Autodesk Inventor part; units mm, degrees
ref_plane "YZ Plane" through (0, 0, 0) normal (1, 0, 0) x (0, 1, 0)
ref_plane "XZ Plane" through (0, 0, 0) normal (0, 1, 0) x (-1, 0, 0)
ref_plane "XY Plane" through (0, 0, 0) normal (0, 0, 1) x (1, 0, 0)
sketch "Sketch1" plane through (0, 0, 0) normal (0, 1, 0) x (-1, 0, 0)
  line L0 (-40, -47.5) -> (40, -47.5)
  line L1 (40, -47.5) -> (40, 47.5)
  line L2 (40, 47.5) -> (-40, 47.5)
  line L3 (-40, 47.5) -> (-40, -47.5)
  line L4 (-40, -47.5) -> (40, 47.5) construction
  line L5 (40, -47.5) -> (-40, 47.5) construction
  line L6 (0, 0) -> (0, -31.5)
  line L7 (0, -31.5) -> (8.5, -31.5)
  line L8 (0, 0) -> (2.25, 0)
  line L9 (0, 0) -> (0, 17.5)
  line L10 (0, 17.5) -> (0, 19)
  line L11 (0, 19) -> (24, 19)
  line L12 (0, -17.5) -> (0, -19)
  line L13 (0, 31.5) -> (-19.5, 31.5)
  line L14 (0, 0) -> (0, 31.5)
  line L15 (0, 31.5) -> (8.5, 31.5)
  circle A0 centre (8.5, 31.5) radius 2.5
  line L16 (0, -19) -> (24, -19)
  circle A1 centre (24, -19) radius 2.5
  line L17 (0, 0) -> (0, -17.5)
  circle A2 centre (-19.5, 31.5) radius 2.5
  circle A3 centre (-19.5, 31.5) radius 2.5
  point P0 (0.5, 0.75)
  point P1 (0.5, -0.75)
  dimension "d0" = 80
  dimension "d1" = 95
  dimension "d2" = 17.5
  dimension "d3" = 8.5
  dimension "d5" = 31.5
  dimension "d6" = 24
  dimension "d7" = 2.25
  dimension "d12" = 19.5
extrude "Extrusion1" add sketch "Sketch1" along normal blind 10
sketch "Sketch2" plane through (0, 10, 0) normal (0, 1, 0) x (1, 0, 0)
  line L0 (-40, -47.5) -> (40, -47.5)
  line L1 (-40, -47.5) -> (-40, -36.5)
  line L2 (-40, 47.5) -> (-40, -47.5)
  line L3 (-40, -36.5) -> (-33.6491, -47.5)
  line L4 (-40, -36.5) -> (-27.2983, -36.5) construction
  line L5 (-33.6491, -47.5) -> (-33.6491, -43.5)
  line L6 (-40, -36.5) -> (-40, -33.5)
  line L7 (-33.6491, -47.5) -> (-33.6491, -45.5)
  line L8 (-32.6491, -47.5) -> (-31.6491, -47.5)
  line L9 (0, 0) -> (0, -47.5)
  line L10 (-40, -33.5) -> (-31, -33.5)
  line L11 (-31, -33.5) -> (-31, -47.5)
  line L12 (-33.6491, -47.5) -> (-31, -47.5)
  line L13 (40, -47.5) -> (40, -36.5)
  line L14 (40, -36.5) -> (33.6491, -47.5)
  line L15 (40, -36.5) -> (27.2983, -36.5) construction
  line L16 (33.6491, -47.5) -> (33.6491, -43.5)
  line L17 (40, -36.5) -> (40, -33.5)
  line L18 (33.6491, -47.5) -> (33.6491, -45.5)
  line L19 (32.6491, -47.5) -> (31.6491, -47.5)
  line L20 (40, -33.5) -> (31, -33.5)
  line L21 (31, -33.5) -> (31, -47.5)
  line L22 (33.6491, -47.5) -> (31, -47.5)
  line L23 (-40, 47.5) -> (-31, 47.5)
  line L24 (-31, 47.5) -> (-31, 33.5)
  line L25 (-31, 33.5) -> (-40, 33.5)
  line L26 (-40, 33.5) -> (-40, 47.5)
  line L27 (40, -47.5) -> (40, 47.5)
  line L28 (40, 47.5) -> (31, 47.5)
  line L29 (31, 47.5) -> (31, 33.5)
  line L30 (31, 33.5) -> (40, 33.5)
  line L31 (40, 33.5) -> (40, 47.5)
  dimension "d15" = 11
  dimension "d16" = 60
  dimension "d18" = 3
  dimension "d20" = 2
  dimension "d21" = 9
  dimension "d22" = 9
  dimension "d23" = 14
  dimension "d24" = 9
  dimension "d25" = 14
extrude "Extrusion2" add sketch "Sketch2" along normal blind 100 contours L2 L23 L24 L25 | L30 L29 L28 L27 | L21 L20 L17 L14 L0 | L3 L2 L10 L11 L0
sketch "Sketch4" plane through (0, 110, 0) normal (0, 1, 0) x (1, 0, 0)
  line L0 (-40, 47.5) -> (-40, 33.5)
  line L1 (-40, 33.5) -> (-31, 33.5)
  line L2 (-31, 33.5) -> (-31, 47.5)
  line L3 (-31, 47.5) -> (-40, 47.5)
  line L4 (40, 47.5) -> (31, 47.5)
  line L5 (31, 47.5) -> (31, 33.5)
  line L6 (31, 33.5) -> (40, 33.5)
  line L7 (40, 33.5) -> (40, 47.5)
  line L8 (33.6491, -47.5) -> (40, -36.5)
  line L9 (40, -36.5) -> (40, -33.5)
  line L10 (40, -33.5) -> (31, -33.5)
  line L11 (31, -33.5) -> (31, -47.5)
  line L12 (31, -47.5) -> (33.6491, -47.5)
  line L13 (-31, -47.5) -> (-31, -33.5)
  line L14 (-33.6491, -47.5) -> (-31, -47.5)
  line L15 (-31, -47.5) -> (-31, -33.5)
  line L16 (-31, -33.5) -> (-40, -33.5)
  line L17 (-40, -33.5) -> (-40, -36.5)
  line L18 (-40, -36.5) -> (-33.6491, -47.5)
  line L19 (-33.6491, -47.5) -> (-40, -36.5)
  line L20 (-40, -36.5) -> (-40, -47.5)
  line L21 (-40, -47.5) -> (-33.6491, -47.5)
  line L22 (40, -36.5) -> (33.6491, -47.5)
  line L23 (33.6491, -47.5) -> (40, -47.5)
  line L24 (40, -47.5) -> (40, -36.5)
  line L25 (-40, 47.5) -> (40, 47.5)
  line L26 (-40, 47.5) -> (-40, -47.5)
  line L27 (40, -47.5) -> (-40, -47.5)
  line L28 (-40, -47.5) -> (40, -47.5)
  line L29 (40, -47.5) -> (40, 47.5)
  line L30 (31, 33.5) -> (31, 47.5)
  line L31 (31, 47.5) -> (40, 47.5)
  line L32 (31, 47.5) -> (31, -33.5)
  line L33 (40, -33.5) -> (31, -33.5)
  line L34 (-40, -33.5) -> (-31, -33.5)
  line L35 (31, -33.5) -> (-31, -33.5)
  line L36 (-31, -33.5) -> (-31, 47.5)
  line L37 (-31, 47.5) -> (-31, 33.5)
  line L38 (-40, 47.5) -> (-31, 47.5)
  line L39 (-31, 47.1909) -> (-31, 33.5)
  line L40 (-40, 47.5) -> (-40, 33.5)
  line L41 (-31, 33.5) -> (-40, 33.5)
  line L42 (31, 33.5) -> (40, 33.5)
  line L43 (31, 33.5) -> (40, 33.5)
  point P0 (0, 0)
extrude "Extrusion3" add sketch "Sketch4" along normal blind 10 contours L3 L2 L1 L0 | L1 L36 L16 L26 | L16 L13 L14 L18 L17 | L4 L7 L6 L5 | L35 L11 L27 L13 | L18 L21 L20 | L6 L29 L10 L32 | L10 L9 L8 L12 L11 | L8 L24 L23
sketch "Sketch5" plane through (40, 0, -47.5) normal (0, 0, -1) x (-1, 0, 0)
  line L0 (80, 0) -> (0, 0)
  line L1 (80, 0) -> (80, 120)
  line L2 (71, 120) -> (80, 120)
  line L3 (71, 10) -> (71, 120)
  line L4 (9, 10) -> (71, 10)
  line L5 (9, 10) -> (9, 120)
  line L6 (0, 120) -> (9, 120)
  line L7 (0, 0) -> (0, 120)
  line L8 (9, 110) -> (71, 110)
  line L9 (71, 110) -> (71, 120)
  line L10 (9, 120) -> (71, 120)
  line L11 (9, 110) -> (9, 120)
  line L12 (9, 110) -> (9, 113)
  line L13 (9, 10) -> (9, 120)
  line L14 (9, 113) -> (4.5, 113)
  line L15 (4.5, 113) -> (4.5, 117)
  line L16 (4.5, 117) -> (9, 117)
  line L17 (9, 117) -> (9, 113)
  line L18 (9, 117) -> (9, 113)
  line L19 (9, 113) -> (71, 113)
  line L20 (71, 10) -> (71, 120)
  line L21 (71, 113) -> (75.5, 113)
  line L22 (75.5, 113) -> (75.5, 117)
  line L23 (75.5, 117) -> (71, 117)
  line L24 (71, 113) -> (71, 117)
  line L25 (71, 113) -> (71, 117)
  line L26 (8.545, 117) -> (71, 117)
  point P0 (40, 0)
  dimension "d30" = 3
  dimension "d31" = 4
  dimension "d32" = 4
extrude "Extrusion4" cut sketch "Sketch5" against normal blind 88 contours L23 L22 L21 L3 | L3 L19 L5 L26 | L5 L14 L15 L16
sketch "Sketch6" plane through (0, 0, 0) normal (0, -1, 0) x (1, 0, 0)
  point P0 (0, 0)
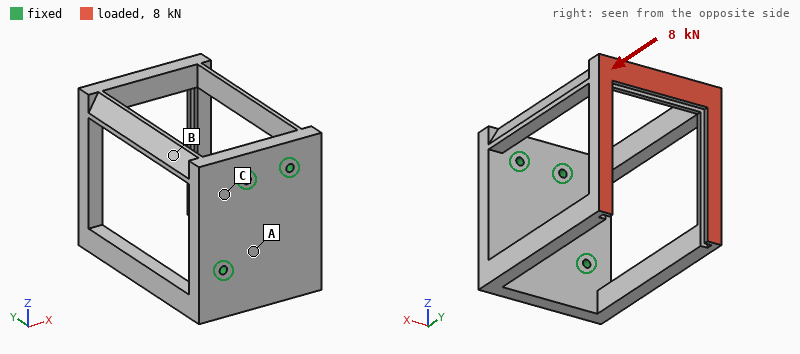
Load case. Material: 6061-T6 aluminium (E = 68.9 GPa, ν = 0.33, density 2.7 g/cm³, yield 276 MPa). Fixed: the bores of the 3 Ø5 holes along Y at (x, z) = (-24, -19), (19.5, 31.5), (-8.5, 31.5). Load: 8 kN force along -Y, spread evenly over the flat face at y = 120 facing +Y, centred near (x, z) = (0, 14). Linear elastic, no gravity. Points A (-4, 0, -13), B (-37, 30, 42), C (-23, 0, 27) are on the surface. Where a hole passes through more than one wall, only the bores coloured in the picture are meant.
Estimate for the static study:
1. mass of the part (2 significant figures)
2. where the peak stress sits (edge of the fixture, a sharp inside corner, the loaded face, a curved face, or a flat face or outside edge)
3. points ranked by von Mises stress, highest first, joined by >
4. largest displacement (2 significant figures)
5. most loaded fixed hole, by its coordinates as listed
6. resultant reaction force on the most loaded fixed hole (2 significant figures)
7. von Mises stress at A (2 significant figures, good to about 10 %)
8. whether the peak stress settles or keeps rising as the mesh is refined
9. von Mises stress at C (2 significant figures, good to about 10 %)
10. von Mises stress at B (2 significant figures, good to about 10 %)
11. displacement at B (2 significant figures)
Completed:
380 g
edge of the fixture
C > A > B
0.36 mm
(19.5, 31.5)
3.3 kN
35 MPa
keeps rising
50 MPa
12 MPa
0.14 mm
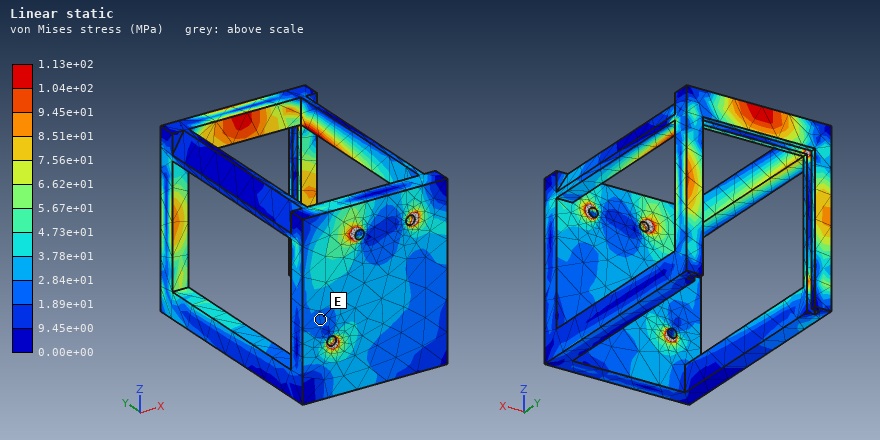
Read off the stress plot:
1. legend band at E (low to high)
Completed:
1.89e+01 to 2.84e+01 MPa
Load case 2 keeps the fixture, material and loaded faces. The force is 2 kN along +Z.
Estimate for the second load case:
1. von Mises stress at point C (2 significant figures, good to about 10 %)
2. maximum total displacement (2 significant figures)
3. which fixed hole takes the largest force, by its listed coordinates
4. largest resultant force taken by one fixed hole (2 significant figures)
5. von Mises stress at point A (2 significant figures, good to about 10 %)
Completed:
37 MPa
1.4 mm
(-24, -19)
2.7 kN
40 MPa
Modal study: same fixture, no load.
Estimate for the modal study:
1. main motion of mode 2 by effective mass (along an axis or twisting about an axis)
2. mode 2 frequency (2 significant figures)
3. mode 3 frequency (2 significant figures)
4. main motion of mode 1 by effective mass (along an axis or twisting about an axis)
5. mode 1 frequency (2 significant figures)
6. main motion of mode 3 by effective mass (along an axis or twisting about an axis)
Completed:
along Z
650 Hz
810 Hz
along X
450 Hz
twisting about Y
